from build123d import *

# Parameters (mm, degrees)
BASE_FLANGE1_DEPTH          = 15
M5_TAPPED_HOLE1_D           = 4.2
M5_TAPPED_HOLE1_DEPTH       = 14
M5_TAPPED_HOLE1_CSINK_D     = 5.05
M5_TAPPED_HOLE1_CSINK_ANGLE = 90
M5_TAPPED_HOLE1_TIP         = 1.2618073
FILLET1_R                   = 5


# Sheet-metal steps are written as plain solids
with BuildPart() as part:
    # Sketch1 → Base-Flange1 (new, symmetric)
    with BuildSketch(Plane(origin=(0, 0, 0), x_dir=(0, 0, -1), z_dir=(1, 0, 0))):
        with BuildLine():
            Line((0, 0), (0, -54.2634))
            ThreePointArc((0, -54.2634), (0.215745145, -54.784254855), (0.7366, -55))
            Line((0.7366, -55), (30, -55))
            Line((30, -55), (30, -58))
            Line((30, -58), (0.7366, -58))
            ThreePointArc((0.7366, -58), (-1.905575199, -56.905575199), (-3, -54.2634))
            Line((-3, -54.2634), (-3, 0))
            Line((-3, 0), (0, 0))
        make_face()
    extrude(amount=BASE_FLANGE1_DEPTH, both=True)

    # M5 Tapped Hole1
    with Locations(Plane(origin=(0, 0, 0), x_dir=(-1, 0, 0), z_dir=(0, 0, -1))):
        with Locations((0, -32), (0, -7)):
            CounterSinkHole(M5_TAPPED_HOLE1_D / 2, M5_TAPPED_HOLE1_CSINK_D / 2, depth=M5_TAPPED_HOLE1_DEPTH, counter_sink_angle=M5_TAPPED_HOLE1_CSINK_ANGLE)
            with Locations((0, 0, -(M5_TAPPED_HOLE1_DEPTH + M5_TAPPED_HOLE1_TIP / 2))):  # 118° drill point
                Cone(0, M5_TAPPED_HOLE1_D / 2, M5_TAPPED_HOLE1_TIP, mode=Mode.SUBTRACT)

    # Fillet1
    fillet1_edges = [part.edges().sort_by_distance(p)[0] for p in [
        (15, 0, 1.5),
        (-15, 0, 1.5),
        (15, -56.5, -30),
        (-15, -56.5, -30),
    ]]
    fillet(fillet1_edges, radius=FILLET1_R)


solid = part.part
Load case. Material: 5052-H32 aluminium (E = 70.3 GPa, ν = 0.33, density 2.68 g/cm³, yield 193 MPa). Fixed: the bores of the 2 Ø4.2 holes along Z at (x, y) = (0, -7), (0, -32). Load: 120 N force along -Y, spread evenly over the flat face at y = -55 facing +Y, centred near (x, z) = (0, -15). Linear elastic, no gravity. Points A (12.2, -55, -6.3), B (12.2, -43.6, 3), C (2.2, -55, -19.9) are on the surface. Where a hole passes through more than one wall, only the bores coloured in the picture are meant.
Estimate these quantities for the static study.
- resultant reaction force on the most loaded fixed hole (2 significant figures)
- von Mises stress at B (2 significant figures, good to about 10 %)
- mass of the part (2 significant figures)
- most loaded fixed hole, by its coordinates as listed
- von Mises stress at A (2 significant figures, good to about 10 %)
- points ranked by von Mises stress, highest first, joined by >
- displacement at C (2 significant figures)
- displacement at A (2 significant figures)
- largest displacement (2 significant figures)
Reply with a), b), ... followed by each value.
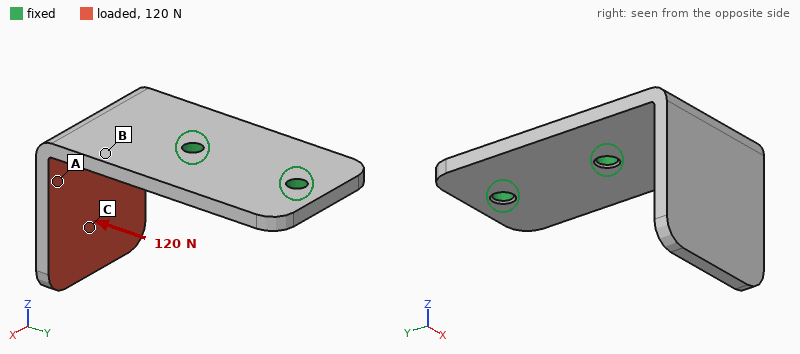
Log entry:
a) 89 N
b) 43 MPa
c) 21 g
d) (0, -32)
e) 23 MPa
f) B > A > C
g) 0.29 mm
h) 0.14 mm
i) 0.43 mm
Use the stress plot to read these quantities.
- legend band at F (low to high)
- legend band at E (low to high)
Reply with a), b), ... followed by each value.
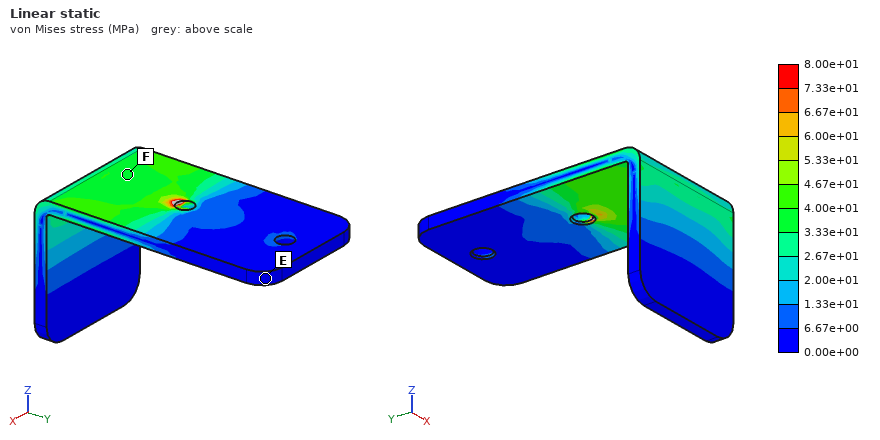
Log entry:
a) 3.33e+01 to 4.00e+01 MPa
b) 0.00e+00 to 6.67e+00 MPa
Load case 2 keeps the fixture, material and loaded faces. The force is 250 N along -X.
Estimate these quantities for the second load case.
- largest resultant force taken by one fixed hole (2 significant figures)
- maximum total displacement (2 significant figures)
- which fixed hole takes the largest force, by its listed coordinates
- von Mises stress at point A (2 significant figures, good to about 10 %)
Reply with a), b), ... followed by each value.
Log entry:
a) 430 N
b) 0.46 mm
c) (0, -32)
d) 33 MPa
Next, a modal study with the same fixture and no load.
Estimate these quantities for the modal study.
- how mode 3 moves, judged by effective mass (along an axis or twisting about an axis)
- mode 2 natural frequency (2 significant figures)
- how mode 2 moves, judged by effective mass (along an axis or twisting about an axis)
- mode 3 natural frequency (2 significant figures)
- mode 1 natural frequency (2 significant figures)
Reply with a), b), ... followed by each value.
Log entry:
a) along Z
b) 1600 Hz
c) along X
d) 2900 Hz
e) 1100 Hz
